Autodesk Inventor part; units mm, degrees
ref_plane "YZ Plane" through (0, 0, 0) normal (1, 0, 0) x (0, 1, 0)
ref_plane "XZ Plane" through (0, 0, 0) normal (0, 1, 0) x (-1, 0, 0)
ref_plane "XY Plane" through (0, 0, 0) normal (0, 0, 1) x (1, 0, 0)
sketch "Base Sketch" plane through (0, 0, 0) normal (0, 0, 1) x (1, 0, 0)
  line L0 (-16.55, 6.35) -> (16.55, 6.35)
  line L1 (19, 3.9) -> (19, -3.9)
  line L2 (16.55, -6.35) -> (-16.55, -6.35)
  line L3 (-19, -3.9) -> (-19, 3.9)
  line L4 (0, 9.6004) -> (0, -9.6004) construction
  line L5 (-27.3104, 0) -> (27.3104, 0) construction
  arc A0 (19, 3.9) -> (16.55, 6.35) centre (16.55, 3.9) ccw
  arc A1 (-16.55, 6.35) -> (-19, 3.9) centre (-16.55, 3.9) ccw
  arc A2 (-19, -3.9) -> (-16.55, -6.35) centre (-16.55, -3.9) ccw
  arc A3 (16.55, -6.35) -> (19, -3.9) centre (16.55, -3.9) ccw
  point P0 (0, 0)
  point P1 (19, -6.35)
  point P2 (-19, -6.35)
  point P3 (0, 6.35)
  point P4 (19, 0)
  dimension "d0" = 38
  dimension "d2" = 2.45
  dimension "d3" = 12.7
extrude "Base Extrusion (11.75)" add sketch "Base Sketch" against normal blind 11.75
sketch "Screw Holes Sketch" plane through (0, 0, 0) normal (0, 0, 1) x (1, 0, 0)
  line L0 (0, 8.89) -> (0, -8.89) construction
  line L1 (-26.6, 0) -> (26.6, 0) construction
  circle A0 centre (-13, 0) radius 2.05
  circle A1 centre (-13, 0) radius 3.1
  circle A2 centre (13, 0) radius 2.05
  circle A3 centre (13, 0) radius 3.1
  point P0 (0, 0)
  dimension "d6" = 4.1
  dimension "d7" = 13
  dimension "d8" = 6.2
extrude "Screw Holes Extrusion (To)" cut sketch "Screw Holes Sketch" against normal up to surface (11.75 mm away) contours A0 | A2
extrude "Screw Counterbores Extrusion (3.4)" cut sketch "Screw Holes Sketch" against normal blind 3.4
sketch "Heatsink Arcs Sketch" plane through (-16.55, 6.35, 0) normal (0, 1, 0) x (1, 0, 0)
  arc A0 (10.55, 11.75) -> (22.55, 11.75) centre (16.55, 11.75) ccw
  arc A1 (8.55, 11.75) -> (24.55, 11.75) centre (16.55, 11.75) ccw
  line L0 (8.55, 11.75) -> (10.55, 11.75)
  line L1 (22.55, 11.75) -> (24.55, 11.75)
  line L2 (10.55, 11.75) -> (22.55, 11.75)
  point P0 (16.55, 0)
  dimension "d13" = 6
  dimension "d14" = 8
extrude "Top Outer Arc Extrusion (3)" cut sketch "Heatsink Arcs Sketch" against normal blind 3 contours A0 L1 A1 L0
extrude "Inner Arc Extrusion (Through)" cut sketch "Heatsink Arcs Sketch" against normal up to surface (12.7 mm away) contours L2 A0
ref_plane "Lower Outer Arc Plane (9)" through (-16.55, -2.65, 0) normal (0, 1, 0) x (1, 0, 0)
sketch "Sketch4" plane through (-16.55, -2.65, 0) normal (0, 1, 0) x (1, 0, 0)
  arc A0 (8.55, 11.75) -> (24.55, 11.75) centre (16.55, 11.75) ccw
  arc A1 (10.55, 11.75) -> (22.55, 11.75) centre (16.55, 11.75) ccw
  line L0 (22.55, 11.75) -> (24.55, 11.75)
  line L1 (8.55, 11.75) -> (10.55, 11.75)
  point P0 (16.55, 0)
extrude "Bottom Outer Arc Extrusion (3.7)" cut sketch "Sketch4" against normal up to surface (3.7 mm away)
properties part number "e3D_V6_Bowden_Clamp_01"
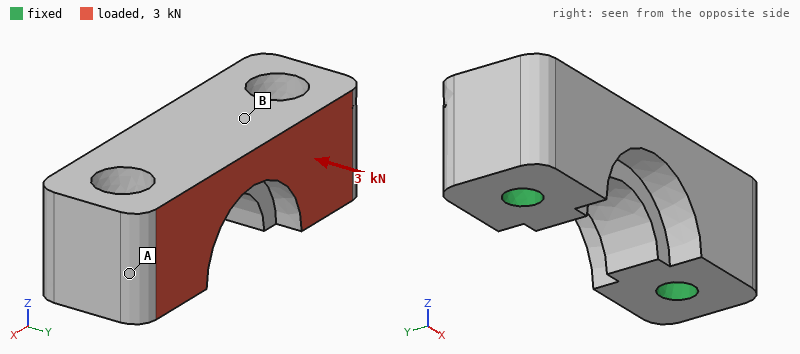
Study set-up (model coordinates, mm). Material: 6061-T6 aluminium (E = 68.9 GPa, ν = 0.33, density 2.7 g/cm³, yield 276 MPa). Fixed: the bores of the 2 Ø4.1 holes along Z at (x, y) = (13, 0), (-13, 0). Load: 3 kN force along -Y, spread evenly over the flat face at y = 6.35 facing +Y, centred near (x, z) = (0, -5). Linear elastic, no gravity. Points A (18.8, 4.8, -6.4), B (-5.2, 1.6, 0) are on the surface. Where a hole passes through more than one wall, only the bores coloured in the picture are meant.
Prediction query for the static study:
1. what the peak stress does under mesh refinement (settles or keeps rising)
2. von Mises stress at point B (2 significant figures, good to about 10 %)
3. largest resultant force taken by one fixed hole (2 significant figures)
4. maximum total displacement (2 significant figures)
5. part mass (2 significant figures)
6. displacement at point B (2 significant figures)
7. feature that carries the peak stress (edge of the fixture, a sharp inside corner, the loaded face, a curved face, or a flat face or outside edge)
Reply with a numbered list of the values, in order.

1. keeps rising
2. 15 MPa
3. 1.5 kN
4. 8.1 µm
5. 11 g
6. 5.8 µm
7. edge of the fixture
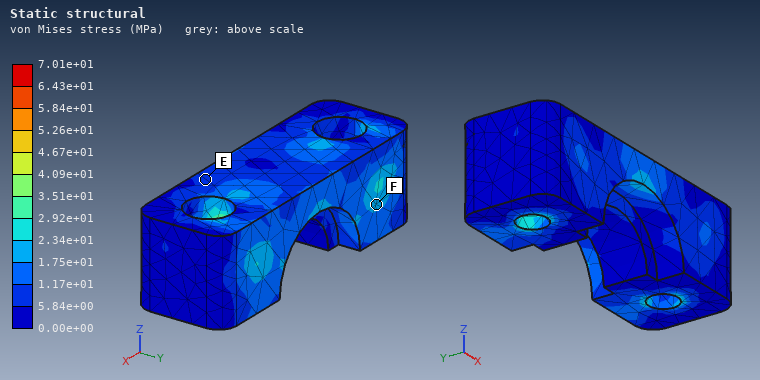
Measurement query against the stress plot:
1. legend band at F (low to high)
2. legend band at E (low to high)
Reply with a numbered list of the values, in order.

1. 1.75e+01 to 2.34e+01 MPa
2. 5.84e+00 to 1.17e+01 MPa
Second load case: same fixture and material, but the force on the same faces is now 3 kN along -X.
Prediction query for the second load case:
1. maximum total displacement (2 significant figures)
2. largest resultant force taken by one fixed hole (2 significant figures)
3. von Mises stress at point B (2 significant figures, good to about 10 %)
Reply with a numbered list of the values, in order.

1. 4.9 µm
2. 1.6 kN
3. 11 MPa
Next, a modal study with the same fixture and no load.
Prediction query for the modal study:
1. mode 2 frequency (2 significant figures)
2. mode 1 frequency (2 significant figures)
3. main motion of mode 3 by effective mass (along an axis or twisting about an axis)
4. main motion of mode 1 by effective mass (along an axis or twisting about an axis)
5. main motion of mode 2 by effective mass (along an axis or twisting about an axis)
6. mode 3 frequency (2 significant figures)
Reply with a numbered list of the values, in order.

1. 51 kHz
2. 38 kHz
3. twisting about X
4. along Y
5. along Z
6. 60 kHz
